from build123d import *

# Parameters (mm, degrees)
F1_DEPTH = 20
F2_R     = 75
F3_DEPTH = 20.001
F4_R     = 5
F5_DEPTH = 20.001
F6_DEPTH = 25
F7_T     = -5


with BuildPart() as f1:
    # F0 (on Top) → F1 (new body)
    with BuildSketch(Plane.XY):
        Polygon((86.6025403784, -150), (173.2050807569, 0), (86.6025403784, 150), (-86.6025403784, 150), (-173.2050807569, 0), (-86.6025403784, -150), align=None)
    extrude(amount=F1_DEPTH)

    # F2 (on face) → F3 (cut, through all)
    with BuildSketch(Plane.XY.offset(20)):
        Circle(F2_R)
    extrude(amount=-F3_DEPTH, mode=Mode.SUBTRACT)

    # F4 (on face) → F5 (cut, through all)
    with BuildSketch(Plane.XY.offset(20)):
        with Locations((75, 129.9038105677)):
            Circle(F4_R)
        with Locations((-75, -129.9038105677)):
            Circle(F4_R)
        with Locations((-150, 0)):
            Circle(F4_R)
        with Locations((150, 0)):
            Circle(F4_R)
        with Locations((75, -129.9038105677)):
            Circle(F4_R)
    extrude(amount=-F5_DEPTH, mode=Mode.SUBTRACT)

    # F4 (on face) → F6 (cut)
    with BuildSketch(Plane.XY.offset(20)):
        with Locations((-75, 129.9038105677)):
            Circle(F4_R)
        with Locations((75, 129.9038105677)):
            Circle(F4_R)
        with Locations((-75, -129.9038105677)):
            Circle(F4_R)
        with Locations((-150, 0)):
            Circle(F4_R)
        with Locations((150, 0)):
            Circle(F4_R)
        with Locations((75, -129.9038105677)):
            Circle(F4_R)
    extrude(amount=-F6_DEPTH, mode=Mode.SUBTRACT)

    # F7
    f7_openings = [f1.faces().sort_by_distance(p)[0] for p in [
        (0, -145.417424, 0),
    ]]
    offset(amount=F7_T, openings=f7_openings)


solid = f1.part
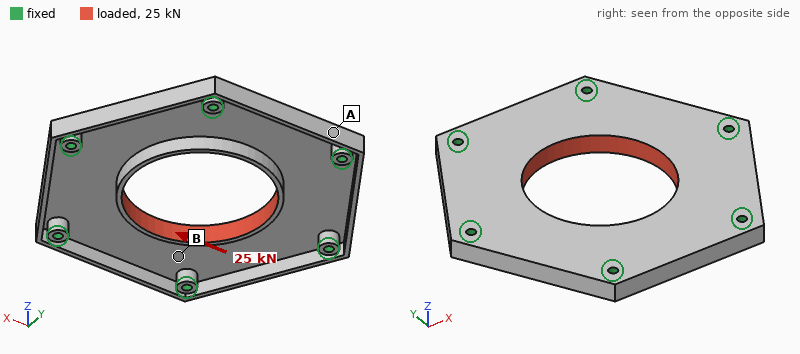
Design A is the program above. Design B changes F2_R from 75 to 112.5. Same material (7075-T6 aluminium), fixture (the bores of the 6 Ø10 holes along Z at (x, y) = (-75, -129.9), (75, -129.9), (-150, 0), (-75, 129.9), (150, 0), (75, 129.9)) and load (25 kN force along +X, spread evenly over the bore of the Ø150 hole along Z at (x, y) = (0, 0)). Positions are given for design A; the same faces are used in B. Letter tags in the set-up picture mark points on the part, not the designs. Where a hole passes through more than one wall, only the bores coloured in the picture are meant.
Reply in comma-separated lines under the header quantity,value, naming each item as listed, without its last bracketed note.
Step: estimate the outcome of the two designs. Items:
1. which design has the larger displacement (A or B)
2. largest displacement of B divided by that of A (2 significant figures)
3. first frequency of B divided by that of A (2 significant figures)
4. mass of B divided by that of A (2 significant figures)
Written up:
quantity,value
which design has the larger displacement,A
largest displacement of B divided by that of A,0.58
first frequency of B divided by that of A,2.3
mass of B divided by that of A,0.79
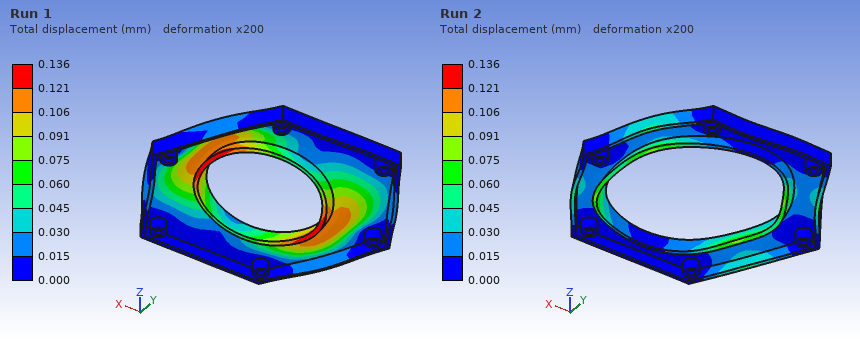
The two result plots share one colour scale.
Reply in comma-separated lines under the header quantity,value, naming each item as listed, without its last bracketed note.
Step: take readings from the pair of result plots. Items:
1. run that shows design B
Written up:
quantity,value
run that shows design B,Run 2
